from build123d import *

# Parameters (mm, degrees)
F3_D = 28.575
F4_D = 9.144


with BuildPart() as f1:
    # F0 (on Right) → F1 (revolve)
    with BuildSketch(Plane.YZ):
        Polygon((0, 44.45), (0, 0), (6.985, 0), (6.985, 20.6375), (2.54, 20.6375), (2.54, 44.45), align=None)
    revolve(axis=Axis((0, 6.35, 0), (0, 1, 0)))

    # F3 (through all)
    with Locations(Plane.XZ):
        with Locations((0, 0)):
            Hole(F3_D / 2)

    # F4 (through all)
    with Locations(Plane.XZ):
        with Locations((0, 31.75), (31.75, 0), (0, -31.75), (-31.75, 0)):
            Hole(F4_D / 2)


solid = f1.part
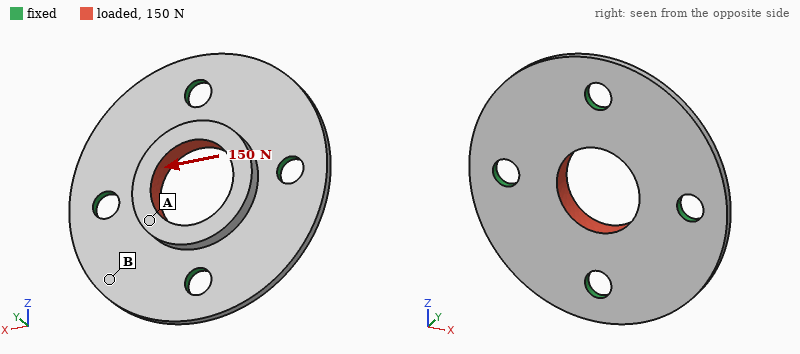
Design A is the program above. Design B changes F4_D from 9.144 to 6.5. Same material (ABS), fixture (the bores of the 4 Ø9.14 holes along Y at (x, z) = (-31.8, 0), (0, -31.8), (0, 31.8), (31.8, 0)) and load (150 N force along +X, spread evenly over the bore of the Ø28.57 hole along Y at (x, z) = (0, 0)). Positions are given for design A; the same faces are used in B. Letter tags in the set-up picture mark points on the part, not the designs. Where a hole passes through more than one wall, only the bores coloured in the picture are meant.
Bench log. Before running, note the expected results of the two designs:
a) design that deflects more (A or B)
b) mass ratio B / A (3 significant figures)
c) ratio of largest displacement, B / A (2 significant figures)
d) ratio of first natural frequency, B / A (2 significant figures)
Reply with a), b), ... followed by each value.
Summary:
a) B
b) 1.02
c) 1.2
d) 0.88
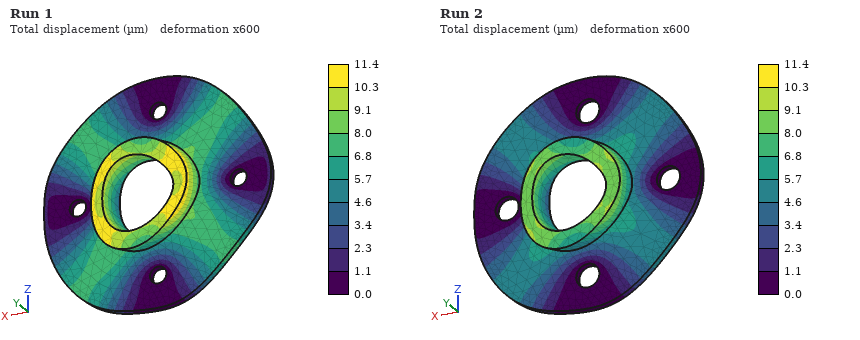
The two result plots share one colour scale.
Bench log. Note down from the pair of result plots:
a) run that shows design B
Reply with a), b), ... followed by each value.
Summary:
a) Run 1
